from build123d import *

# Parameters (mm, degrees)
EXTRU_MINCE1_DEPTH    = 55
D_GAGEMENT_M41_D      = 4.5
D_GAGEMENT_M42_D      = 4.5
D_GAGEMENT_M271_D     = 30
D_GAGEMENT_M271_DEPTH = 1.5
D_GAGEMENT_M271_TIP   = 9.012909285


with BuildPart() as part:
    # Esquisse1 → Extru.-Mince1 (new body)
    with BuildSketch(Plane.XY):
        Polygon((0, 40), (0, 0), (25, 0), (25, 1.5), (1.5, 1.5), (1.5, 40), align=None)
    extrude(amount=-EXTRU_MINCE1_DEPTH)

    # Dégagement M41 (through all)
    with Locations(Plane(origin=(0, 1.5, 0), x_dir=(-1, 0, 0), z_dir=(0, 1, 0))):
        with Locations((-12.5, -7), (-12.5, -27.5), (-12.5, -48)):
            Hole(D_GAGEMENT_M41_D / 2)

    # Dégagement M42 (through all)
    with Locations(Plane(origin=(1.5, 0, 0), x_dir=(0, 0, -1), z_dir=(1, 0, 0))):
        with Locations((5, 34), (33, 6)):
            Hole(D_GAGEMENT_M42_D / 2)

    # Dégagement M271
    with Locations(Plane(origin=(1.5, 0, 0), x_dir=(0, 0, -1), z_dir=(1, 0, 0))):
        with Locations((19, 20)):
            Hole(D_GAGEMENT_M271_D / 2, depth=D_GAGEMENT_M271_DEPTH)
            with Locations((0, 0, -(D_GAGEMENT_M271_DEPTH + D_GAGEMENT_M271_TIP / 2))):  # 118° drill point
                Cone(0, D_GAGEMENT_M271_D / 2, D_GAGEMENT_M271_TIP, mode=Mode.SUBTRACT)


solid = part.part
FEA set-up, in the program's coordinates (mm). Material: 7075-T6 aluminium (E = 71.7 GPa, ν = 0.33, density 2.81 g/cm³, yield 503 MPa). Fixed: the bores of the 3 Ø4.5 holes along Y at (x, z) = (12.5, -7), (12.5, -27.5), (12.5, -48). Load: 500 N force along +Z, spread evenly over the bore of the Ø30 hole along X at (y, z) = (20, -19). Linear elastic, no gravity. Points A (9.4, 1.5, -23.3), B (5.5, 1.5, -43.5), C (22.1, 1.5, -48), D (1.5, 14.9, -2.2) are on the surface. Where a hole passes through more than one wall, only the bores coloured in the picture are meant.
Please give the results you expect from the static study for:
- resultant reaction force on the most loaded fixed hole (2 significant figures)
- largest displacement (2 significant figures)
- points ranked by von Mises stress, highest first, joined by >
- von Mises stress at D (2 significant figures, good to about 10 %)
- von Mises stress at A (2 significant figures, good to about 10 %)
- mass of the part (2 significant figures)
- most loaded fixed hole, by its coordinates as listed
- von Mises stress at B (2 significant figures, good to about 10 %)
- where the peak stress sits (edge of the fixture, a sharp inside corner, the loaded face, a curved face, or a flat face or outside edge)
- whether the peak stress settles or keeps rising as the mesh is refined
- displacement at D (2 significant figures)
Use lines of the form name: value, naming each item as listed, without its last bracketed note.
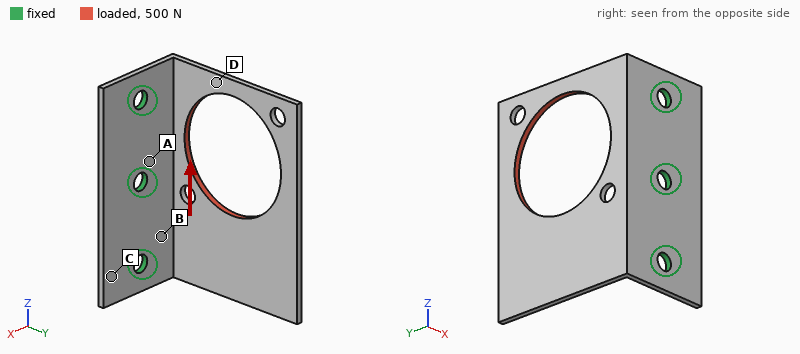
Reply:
resultant reaction force on the most loaded fixed hole: 330 N
largest displacement: 0.74 mm
points ranked by von Mises stress, highest first, joined by >: B > D > A > C
von Mises stress at D: 91 MPa
von Mises stress at A: 54 MPa
mass of the part: 11 g
most loaded fixed hole, by its coordinates as listed: (12.5, -7)
von Mises stress at B: 120 MPa
where the peak stress sits: edge of the fixture
whether the peak stress settles or keeps rising as the mesh is refined: keeps rising
displacement at D: 0.35 mm
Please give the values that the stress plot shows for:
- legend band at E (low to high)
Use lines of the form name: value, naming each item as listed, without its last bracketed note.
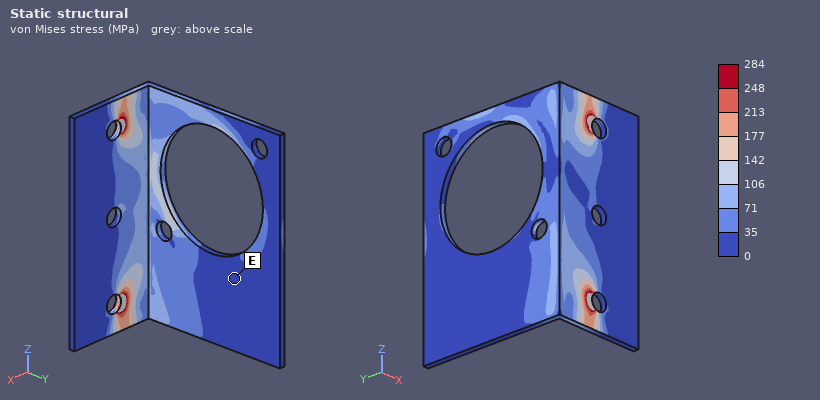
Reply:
legend band at E: 0 to 35 MPa
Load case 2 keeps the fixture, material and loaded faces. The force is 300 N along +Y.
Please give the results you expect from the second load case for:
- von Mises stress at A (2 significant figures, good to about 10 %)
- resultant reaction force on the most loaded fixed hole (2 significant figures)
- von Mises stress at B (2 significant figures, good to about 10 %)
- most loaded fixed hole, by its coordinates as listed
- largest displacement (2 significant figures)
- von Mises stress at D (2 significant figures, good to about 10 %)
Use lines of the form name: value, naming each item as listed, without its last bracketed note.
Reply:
von Mises stress at A: 110 MPa
resultant reaction force on the most loaded fixed hole: 160 N
von Mises stress at B: 44 MPa
most loaded fixed hole, by its coordinates as listed: (12.5, -7)
largest displacement: 0.69 mm
von Mises stress at D: 32 MPa
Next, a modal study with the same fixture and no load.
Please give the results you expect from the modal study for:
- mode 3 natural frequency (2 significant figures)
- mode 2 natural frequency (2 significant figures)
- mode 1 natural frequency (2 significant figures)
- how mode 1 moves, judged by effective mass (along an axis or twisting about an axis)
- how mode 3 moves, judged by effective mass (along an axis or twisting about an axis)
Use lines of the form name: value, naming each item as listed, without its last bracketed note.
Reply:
mode 3 natural frequency: 2400 Hz
mode 2 natural frequency: 1100 Hz
mode 1 natural frequency: 550 Hz
how mode 1 moves, judged by effective mass: along X
how mode 3 moves, judged by effective mass: along Z
